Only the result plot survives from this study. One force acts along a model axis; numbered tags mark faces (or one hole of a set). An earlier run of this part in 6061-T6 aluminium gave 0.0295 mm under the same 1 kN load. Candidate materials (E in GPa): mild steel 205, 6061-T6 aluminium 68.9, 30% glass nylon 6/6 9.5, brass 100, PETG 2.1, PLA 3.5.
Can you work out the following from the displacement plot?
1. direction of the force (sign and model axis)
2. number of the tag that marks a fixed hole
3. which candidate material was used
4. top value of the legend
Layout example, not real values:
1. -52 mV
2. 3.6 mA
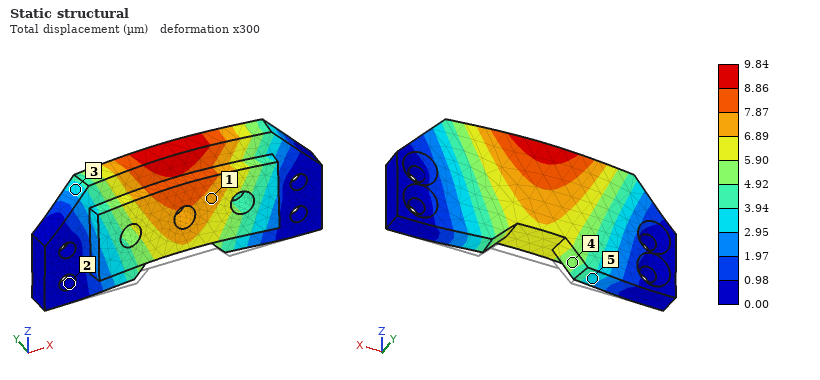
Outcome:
1. +Y
2. 2
3. mild steel
4. 9.84 µm
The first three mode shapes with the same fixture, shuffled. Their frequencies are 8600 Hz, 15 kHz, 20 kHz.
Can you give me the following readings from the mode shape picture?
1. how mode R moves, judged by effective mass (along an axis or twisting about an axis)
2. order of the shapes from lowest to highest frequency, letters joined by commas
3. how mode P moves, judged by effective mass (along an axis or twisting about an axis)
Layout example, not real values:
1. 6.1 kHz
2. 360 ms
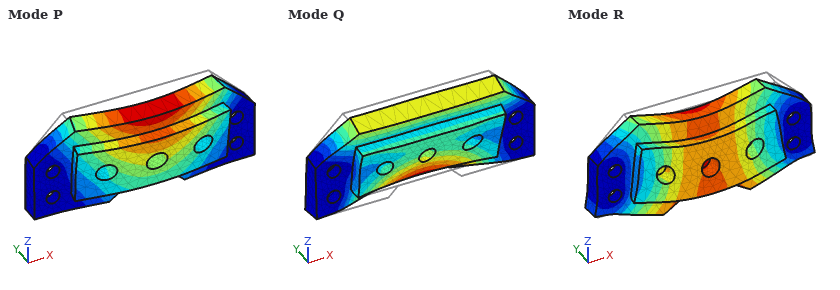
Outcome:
1. along Z
2. P, Q, R
3. along Y
